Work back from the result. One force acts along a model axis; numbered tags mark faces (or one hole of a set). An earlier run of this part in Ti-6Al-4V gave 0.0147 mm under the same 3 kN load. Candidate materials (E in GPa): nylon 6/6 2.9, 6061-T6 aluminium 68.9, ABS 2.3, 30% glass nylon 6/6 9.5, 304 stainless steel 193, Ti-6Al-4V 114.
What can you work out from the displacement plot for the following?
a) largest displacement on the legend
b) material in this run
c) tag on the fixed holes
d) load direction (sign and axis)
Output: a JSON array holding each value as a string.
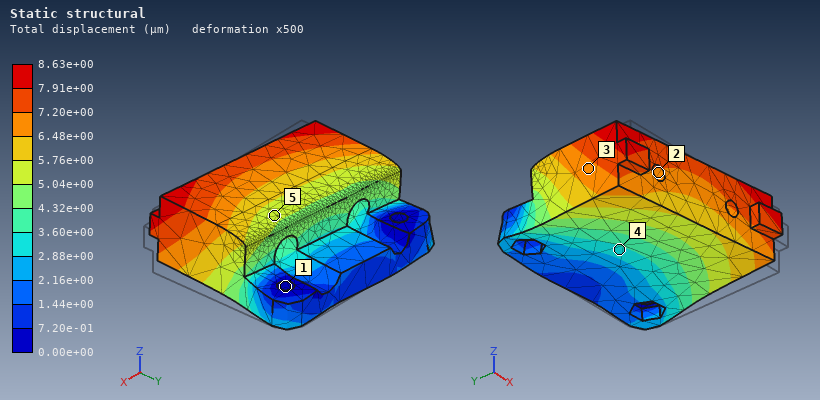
["8.63e+00 µm", "304 stainless steel", "1", "-X"]
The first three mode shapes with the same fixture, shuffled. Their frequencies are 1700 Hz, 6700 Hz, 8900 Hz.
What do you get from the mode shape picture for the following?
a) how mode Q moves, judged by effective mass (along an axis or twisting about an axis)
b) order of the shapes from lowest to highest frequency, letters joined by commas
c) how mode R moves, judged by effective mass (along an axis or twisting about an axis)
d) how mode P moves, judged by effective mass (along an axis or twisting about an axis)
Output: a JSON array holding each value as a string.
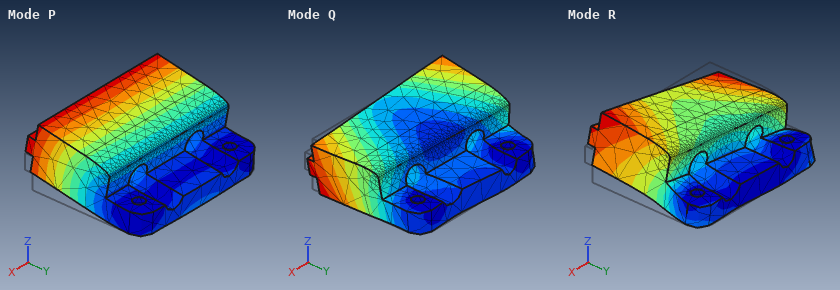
["along X", "P, R, Q", "along X", "along Z"]
